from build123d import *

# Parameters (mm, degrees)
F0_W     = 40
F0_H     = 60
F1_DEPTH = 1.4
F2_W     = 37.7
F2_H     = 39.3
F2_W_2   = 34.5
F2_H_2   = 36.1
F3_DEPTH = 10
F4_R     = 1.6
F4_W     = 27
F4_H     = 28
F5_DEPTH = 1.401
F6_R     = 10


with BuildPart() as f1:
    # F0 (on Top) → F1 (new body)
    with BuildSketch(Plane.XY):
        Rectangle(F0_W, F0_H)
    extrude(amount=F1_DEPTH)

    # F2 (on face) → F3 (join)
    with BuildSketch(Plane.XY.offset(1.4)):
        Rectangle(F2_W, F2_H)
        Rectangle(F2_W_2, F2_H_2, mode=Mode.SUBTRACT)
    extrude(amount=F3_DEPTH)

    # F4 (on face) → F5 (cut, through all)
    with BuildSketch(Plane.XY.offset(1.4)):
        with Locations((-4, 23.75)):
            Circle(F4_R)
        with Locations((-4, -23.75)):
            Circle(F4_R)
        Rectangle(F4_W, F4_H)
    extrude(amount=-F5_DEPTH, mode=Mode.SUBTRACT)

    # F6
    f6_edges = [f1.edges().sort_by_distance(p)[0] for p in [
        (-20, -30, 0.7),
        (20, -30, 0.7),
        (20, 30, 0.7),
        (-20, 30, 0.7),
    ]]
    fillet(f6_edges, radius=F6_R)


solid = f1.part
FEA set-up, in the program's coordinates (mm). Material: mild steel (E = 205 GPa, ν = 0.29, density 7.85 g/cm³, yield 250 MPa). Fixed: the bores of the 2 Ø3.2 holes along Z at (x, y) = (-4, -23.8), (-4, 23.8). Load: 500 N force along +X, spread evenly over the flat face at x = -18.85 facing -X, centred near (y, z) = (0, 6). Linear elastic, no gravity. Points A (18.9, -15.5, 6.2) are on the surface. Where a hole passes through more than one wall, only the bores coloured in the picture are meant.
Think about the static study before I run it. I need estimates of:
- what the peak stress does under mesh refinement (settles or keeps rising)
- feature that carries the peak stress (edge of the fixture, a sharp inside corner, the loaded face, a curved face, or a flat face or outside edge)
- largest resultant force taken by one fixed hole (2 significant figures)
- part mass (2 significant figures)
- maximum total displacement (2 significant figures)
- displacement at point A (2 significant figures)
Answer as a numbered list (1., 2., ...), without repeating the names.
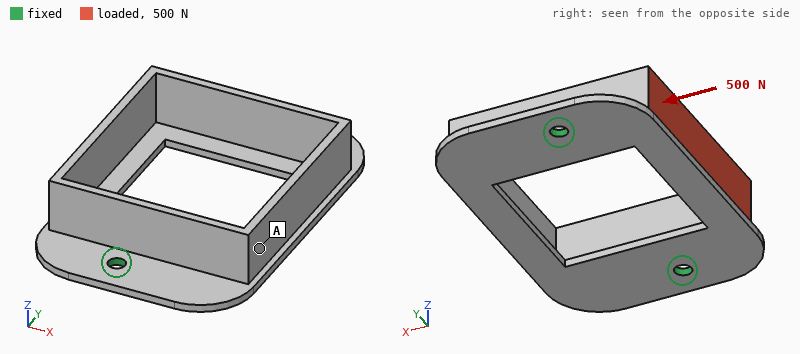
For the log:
1. keeps rising
2. edge of the fixture
3. 270 N
4. 35 g
5. 0.10 mm
6. 0.066 mm
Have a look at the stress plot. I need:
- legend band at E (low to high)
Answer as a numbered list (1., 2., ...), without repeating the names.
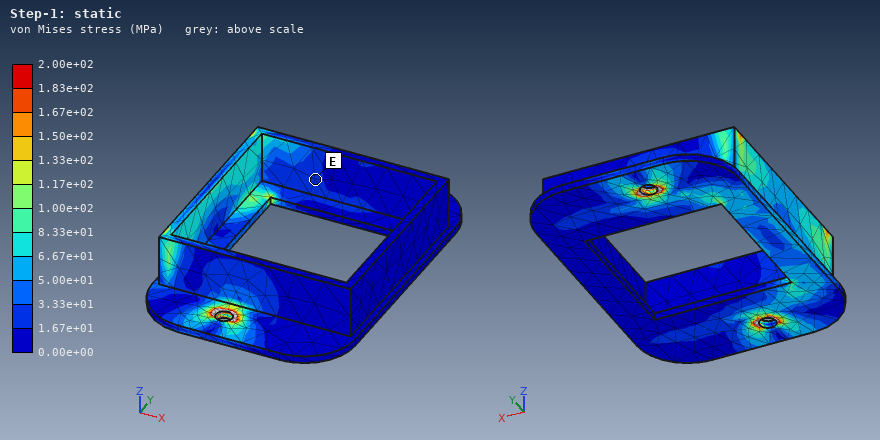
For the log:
1. 1.67e+01 to 3.33e+01 MPa
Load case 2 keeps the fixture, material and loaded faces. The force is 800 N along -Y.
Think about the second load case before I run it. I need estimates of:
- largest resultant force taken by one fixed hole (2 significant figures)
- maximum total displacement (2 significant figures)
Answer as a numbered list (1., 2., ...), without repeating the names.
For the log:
1. 440 N
2. 37 µm
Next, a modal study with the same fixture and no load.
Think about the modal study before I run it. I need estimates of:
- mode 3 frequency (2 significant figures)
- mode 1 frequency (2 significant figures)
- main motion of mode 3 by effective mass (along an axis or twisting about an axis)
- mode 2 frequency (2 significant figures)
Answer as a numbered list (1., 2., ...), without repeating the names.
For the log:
1. 6500 Hz
2. 1800 Hz
3. along Z
4. 3300 Hz
